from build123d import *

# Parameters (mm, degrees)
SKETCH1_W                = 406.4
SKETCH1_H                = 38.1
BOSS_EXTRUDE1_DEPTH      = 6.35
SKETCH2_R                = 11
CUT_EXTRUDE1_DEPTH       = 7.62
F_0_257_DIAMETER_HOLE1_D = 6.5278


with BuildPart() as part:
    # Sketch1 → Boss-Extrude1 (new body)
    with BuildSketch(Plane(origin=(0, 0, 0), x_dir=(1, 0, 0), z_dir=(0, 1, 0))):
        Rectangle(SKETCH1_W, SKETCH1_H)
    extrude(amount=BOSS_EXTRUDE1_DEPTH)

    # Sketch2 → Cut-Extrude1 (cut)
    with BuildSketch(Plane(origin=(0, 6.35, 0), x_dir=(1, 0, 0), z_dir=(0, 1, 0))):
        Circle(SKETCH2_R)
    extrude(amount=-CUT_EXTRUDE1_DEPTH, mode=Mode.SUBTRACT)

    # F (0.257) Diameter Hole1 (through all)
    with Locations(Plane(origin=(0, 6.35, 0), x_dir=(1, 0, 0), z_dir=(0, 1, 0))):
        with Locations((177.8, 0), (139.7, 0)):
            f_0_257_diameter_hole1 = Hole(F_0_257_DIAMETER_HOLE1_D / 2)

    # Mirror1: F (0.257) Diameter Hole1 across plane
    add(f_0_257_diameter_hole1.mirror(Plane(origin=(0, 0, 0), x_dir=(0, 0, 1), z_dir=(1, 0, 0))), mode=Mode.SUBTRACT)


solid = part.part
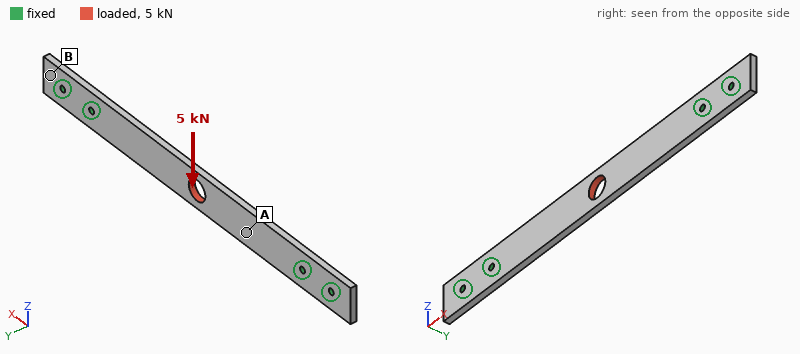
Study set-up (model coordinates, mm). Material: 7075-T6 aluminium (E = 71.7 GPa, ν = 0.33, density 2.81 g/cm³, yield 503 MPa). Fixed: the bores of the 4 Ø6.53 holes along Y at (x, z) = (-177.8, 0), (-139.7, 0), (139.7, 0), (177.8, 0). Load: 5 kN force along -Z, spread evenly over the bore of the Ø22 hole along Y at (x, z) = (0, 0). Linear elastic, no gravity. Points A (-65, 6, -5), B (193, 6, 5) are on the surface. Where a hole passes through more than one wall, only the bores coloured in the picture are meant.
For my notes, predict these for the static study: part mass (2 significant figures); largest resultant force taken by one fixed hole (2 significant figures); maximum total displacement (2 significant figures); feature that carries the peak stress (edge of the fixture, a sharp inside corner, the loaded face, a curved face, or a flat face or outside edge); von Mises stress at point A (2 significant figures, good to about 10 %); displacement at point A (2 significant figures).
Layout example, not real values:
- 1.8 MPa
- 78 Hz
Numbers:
- 270 g
- 5.7 kN
- 0.44 mm
- edge of the fixture
- 26 MPa
- 0.26 mm
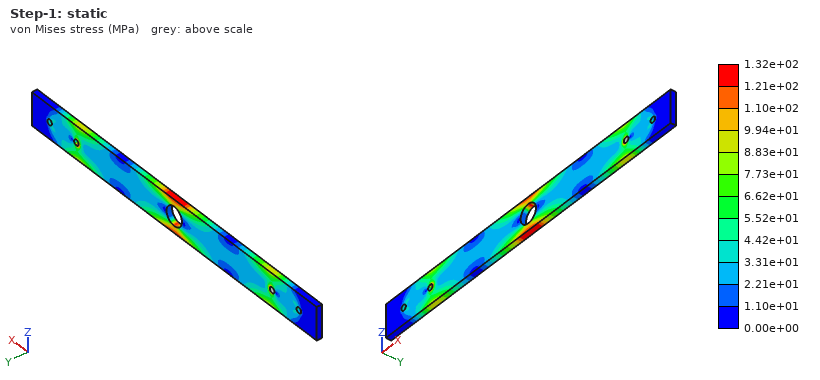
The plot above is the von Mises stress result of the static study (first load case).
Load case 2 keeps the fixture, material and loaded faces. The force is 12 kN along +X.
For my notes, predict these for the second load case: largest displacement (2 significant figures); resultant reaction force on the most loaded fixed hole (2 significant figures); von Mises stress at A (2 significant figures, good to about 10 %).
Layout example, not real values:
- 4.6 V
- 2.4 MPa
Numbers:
- 52 µm
- 4.9 kN
- 25 MPa
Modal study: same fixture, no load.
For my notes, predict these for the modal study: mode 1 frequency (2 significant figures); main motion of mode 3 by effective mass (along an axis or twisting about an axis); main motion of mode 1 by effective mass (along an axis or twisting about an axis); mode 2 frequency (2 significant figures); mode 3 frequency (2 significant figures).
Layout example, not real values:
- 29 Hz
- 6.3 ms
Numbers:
- 420 Hz
- twisting about X
- along Y
- 1200 Hz
- 1800 Hz
